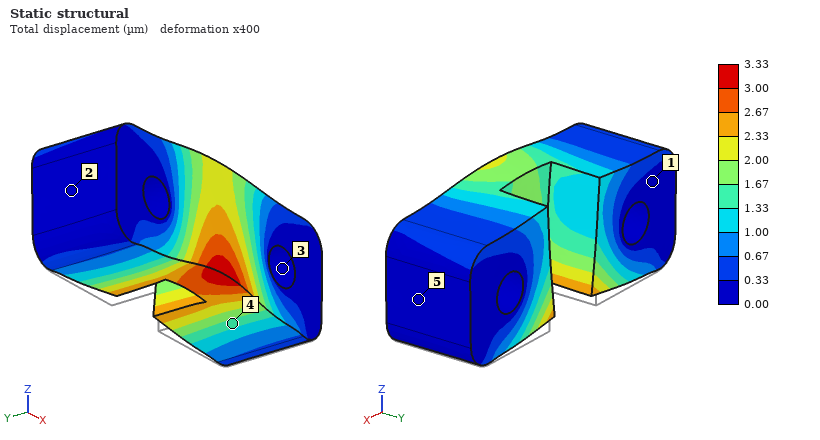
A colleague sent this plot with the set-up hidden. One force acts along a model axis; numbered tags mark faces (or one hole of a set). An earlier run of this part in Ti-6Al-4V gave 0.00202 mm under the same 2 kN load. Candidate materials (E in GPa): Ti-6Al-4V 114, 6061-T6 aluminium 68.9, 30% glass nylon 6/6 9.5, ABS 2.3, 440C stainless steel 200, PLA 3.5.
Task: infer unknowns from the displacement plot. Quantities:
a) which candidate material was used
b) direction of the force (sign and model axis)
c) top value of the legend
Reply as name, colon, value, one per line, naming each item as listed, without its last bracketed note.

which candidate material was used: 6061-T6 aluminium
direction of the force: +Z
top value of the legend: 3.33 µm
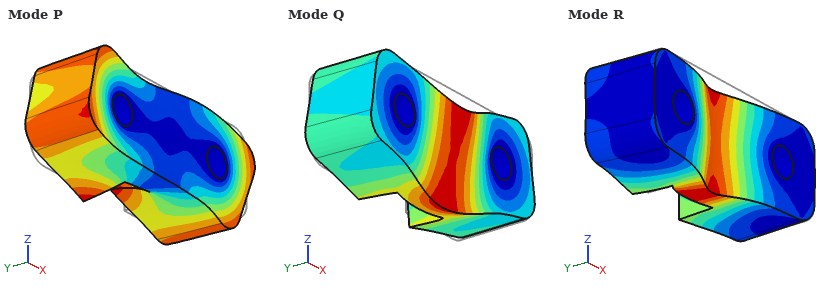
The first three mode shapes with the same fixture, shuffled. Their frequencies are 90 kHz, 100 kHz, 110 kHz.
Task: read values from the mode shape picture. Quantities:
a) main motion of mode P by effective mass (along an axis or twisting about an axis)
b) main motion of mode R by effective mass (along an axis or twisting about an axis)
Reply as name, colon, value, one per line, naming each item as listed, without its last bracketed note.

main motion of mode P by effective mass: twisting about Y
main motion of mode R by effective mass: along Y
